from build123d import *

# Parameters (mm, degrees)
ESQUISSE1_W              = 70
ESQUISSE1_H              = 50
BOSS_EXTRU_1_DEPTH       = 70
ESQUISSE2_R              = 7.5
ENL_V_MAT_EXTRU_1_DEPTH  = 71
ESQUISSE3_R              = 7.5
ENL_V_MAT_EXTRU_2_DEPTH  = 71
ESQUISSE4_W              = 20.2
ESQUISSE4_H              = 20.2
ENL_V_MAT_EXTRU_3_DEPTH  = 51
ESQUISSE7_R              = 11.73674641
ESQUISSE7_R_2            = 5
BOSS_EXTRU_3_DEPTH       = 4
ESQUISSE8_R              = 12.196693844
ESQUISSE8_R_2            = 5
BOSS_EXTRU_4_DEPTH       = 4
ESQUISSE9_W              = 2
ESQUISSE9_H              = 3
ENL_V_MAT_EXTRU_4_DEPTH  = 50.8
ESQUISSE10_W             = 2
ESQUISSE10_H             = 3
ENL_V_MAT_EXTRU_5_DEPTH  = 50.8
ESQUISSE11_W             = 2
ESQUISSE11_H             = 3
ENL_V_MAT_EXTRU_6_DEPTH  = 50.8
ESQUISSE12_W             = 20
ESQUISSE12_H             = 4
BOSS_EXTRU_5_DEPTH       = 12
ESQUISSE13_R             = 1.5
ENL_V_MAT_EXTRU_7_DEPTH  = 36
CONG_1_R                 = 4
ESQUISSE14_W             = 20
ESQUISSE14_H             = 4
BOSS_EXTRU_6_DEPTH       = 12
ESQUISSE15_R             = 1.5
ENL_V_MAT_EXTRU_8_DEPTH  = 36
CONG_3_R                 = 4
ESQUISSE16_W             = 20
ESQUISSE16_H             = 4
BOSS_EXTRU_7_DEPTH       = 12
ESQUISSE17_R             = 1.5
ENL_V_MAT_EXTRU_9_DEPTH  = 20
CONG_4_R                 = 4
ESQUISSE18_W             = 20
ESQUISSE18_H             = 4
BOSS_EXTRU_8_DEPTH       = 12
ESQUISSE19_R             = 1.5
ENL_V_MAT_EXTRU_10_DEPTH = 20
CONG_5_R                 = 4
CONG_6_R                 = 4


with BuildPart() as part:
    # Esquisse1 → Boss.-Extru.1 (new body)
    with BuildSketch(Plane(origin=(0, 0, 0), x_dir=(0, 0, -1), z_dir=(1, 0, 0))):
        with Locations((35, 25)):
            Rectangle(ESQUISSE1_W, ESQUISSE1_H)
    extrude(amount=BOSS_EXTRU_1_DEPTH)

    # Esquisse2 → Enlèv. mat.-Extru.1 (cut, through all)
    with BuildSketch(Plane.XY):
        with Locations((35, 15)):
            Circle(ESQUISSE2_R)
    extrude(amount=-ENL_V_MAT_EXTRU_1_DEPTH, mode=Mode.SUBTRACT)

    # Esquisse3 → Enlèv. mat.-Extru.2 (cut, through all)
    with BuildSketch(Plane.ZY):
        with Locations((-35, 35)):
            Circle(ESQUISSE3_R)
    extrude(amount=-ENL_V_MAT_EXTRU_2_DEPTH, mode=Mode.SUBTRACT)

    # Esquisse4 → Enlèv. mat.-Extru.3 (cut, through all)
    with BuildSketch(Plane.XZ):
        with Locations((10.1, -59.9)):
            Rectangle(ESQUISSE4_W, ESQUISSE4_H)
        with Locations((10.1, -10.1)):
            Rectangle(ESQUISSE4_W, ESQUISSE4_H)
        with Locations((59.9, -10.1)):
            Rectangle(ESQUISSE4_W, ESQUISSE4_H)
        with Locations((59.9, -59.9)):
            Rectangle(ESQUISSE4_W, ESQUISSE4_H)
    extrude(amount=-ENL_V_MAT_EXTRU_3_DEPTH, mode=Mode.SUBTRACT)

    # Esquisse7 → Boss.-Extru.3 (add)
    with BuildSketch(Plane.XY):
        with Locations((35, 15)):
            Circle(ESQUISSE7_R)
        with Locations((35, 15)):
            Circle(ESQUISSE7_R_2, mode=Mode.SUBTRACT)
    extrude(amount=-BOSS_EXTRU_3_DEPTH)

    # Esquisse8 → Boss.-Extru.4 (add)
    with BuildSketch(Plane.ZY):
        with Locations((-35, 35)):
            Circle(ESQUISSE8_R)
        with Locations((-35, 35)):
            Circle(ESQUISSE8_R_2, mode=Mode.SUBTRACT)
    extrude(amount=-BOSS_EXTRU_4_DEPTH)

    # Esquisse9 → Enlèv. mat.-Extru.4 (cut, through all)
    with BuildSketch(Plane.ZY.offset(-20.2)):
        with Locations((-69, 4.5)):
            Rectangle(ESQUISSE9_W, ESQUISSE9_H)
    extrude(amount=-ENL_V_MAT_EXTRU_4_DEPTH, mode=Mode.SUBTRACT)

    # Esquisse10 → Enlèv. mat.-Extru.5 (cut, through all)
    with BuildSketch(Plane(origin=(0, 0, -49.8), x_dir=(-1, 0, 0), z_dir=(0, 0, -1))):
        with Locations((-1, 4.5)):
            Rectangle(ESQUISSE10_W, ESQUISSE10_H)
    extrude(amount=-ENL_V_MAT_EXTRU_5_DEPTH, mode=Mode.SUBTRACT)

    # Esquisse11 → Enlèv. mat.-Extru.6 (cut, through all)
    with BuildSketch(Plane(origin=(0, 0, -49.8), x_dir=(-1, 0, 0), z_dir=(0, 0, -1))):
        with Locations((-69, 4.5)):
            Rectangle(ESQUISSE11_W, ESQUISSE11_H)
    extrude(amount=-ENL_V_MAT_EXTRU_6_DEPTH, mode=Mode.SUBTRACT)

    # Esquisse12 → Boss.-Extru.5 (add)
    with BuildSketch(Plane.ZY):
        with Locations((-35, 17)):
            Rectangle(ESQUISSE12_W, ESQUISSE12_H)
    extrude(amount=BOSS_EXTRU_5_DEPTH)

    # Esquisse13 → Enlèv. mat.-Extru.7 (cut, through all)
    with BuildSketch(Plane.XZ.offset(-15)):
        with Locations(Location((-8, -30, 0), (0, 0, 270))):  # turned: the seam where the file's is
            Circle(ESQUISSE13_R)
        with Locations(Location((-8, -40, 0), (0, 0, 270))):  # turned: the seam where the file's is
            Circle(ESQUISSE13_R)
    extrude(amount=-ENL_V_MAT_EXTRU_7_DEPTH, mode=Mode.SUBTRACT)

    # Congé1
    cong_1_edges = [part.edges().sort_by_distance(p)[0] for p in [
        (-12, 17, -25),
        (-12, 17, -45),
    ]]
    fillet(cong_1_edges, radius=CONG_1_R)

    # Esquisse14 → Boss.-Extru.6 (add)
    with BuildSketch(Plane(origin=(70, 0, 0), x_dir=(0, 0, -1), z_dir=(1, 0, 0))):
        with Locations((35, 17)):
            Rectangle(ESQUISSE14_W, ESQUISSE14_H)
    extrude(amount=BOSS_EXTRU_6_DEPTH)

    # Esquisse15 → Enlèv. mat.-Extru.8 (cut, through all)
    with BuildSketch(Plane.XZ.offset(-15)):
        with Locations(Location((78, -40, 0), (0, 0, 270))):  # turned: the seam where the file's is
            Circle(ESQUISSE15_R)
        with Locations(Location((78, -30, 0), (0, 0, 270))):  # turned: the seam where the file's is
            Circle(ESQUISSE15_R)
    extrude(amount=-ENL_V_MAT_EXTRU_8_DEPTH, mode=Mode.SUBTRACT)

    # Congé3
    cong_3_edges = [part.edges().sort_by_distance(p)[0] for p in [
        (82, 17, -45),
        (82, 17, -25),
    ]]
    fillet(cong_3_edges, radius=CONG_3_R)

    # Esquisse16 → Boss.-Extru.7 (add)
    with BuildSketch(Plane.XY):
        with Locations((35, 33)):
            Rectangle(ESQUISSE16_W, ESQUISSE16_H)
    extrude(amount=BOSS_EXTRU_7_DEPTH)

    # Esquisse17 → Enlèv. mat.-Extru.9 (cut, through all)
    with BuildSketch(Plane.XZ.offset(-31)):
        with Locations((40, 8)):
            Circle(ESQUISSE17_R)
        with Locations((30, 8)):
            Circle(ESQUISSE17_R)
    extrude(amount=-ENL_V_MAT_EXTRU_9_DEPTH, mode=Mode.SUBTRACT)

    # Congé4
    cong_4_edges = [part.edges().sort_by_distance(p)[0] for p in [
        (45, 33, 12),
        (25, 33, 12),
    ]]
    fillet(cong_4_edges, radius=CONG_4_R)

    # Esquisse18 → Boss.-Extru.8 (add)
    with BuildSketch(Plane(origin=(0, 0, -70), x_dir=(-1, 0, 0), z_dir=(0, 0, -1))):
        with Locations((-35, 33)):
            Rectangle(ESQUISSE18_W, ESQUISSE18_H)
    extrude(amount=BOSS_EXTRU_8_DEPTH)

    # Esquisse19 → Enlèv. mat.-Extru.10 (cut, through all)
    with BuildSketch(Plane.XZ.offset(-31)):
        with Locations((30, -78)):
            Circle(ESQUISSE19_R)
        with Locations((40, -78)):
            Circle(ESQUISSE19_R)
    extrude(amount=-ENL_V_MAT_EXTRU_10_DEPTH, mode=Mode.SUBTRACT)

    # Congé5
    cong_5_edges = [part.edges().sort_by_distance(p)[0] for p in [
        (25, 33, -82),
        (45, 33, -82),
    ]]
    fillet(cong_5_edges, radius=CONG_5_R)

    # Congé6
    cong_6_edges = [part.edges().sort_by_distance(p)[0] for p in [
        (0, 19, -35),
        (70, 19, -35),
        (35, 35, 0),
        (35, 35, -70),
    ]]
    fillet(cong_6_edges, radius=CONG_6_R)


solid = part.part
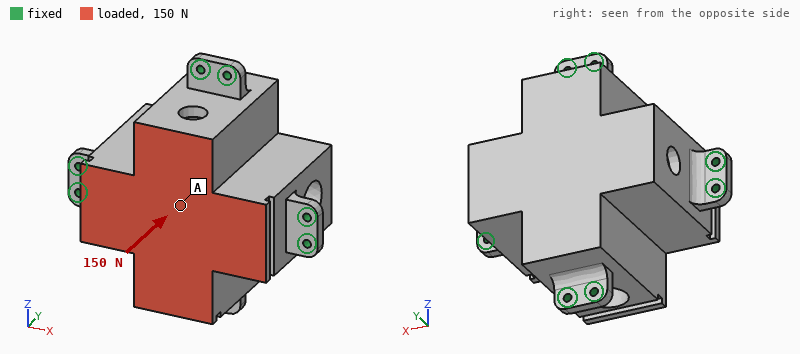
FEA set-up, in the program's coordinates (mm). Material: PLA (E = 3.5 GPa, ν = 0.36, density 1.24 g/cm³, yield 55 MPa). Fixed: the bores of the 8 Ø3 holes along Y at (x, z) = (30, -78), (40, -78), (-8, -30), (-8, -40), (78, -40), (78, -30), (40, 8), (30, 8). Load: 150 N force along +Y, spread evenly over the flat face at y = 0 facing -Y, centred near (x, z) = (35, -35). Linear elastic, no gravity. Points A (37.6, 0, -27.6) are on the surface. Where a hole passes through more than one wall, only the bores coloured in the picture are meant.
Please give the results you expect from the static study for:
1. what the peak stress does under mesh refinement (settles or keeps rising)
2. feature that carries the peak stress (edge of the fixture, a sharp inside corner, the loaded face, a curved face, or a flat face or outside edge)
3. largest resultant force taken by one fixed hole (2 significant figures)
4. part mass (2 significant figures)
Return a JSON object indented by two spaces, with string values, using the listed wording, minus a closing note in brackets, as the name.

{
  "what the peak stress does under mesh refinement": "keeps rising",
  "feature that carries the peak stress": "edge of the fixture",
  "largest resultant force taken by one fixed hole": "19 N",
  "part mass": "180 g"
}
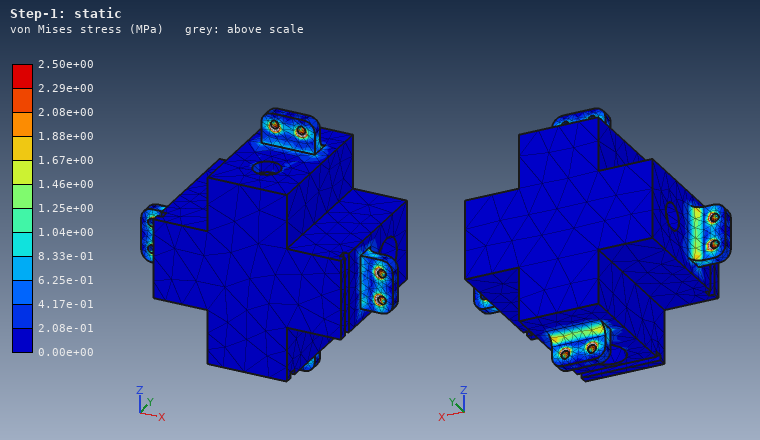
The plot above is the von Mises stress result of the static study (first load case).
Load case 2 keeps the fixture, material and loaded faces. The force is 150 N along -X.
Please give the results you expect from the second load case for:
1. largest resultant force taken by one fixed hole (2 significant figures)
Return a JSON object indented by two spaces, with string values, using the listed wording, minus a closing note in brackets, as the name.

{
  "largest resultant force taken by one fixed hole": "39 N"
}
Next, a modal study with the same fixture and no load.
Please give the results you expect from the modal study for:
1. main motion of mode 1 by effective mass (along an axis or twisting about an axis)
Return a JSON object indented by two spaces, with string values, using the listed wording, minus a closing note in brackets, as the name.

{
  "main motion of mode 1 by effective mass": "along Y"
}
